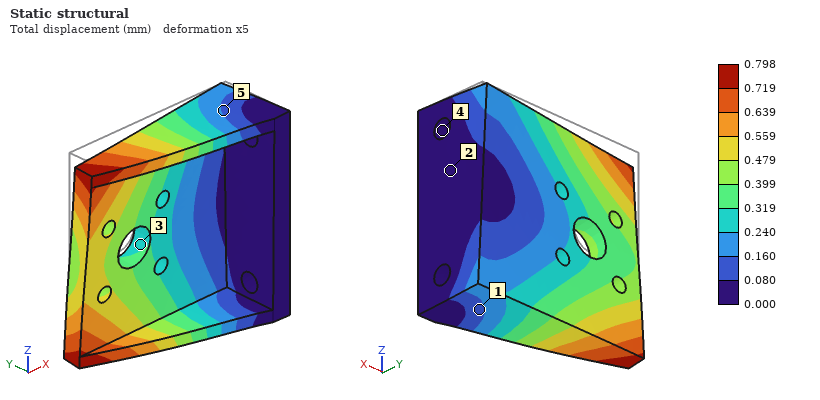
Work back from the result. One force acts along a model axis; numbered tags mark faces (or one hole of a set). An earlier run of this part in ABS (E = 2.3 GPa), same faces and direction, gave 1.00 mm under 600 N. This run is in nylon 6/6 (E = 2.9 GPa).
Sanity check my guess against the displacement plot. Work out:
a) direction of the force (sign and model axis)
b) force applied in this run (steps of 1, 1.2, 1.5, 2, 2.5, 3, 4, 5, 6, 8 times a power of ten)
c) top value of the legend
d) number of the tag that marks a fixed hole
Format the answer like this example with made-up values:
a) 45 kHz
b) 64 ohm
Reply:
a) -Z
b) 600 N
c) 0.798 mm
d) 4
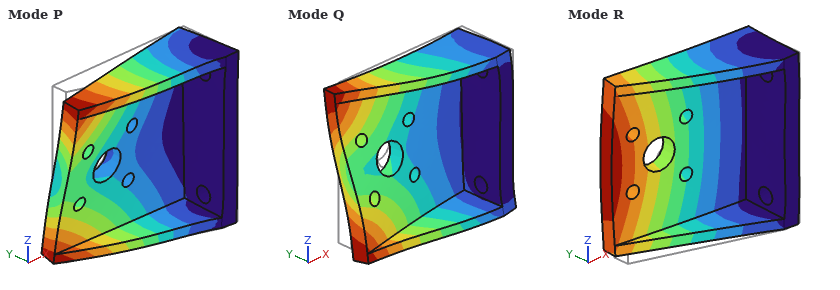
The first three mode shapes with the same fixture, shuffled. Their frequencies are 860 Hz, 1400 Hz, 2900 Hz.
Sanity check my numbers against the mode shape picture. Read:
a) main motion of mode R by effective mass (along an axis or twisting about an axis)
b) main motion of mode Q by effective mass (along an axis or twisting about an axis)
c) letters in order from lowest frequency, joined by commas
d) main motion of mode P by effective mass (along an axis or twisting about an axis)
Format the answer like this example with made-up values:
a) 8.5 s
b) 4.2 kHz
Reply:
a) along Y
b) along Z
c) R, P, Q
d) along Z
